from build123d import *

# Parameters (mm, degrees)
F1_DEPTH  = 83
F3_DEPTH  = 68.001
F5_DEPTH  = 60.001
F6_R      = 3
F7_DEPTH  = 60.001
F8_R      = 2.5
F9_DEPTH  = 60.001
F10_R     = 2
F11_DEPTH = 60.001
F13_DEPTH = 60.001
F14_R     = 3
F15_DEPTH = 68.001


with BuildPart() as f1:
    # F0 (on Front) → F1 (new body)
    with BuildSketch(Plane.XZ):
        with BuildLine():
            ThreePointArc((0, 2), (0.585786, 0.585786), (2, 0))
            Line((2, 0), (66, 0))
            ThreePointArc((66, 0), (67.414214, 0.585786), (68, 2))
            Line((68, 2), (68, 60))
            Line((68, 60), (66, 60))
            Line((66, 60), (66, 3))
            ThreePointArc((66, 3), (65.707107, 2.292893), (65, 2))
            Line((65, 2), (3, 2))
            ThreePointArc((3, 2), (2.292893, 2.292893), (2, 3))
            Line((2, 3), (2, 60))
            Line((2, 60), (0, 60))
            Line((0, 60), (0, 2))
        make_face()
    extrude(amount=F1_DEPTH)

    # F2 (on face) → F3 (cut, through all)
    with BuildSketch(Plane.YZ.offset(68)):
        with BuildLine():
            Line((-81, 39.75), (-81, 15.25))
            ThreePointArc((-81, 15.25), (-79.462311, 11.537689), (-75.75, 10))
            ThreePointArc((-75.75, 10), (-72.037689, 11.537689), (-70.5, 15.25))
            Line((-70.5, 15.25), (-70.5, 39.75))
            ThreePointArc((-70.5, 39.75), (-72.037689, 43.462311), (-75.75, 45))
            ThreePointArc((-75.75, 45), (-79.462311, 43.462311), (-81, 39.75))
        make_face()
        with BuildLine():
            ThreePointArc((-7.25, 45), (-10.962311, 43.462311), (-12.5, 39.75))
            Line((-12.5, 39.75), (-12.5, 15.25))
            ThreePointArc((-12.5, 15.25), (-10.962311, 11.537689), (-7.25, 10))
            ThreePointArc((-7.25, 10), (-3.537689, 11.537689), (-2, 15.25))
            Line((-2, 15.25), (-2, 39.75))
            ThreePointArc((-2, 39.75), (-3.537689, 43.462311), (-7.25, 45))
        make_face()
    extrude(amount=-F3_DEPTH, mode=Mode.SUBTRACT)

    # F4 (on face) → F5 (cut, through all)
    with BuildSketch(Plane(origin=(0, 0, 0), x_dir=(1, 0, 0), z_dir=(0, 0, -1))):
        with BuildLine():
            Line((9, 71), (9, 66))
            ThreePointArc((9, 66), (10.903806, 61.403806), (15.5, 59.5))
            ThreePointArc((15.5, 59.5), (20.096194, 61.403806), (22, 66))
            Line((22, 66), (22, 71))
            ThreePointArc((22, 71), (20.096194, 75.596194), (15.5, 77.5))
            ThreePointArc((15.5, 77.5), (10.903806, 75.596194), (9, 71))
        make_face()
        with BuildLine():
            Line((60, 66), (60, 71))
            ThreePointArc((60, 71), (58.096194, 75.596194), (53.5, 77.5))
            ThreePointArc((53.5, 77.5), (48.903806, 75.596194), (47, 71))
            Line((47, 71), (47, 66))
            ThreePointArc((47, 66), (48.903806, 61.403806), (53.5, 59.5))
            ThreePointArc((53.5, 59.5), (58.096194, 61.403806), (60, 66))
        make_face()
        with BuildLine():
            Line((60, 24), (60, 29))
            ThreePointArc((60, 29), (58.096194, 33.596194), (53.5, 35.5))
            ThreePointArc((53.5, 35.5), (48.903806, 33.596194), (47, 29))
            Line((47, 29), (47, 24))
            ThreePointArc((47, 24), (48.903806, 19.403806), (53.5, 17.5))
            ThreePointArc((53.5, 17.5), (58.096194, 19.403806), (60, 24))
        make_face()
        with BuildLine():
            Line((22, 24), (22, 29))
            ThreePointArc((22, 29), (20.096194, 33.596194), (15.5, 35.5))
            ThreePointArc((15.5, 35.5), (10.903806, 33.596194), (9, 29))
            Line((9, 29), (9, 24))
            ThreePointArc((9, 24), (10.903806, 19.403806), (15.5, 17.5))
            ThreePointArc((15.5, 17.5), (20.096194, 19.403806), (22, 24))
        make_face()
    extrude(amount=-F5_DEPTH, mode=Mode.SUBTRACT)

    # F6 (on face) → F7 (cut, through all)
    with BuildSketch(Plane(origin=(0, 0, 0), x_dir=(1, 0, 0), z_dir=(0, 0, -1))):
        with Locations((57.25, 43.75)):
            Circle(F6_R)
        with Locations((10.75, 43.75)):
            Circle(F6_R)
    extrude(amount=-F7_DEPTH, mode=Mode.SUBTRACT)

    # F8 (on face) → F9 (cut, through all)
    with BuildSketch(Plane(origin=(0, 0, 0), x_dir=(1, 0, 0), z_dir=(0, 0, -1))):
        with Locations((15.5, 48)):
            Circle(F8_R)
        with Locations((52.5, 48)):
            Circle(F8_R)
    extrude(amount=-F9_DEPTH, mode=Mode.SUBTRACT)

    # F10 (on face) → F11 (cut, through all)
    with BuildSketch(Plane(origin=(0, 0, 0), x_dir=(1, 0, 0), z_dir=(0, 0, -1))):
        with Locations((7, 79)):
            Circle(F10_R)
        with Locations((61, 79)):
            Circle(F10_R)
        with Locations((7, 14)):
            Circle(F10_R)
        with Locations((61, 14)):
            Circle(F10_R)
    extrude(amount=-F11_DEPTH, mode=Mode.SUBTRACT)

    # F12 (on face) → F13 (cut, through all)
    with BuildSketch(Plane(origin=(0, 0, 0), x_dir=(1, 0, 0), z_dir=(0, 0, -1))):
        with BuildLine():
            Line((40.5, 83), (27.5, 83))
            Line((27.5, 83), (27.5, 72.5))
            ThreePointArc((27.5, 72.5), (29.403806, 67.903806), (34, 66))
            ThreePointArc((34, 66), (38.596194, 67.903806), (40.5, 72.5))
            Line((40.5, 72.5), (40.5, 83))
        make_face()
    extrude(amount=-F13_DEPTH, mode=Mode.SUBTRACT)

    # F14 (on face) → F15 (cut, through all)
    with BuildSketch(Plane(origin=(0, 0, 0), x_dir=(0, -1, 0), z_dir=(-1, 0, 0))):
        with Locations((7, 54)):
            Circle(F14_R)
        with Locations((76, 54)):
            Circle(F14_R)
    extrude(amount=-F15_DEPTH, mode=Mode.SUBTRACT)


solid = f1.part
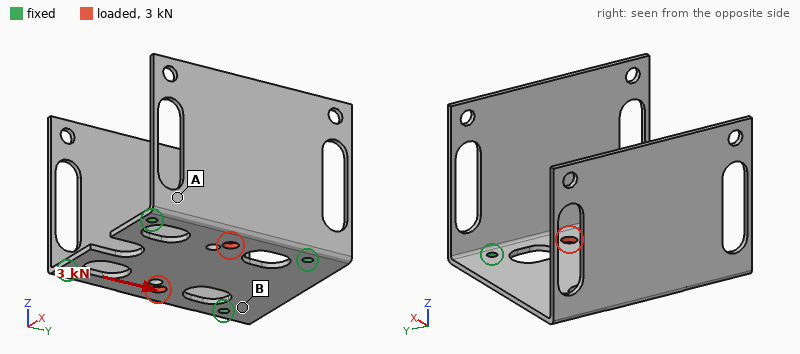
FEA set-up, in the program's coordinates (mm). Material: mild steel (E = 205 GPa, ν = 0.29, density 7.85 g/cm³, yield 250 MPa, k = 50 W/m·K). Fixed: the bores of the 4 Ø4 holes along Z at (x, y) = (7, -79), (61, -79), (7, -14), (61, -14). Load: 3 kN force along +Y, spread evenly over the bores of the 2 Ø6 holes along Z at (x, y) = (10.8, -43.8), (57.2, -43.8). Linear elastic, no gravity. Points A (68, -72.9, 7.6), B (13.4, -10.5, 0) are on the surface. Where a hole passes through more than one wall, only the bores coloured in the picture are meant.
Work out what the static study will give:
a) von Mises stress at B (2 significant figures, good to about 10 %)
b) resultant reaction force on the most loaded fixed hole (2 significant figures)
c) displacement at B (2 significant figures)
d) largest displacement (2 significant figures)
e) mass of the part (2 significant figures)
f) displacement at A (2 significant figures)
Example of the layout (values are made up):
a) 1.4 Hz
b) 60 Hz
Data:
a) 19 MPa
b) 930 N
c) 1.1 µm
d) 7.3 µm
e) 200 g
f) 2.6 µm
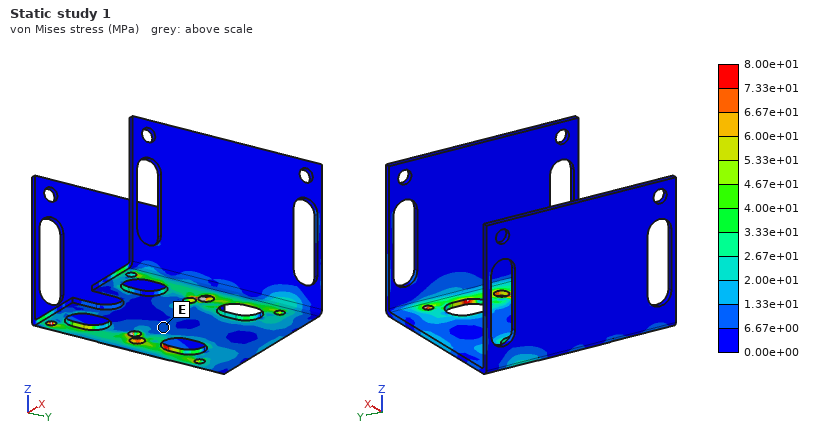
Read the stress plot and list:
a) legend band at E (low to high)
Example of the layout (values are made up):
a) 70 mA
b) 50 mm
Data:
a) 6.67e+00 to 1.33e+01 MPa
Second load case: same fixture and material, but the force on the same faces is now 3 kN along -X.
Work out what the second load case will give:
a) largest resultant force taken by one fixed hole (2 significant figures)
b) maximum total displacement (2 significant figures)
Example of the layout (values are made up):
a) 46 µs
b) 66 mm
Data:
a) 980 N
b) 18 µm
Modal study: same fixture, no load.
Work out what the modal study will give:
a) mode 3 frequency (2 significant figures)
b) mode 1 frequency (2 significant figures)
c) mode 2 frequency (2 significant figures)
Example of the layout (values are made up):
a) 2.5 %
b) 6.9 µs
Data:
a) 880 Hz
b) 370 Hz
c) 380 Hz
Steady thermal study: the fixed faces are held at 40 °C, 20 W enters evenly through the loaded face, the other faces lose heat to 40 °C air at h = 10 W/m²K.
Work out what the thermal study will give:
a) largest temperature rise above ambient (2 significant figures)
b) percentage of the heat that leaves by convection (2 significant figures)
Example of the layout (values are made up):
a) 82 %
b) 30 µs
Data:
a) 74 K
b) 29 %
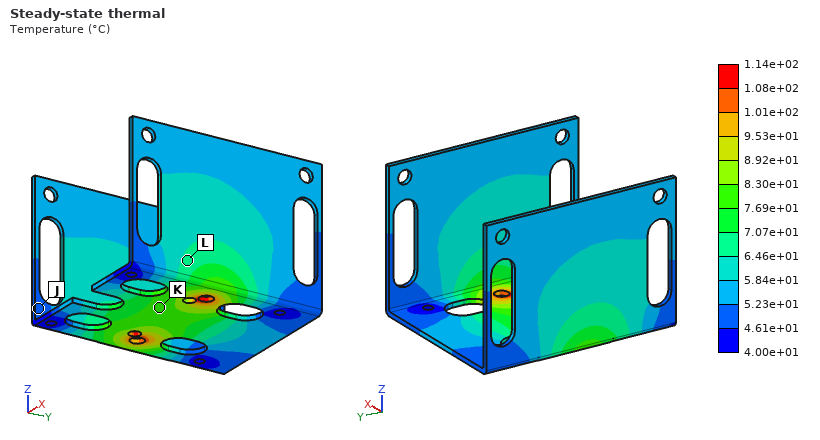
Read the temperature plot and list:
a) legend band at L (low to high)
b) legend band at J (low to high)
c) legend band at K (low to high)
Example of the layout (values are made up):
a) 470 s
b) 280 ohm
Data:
a) 6.46e+01 to 7.07e+01 °C
b) 4.61e+01 to 5.23e+01 °C
c) 7.69e+01 to 8.30e+01 °C
